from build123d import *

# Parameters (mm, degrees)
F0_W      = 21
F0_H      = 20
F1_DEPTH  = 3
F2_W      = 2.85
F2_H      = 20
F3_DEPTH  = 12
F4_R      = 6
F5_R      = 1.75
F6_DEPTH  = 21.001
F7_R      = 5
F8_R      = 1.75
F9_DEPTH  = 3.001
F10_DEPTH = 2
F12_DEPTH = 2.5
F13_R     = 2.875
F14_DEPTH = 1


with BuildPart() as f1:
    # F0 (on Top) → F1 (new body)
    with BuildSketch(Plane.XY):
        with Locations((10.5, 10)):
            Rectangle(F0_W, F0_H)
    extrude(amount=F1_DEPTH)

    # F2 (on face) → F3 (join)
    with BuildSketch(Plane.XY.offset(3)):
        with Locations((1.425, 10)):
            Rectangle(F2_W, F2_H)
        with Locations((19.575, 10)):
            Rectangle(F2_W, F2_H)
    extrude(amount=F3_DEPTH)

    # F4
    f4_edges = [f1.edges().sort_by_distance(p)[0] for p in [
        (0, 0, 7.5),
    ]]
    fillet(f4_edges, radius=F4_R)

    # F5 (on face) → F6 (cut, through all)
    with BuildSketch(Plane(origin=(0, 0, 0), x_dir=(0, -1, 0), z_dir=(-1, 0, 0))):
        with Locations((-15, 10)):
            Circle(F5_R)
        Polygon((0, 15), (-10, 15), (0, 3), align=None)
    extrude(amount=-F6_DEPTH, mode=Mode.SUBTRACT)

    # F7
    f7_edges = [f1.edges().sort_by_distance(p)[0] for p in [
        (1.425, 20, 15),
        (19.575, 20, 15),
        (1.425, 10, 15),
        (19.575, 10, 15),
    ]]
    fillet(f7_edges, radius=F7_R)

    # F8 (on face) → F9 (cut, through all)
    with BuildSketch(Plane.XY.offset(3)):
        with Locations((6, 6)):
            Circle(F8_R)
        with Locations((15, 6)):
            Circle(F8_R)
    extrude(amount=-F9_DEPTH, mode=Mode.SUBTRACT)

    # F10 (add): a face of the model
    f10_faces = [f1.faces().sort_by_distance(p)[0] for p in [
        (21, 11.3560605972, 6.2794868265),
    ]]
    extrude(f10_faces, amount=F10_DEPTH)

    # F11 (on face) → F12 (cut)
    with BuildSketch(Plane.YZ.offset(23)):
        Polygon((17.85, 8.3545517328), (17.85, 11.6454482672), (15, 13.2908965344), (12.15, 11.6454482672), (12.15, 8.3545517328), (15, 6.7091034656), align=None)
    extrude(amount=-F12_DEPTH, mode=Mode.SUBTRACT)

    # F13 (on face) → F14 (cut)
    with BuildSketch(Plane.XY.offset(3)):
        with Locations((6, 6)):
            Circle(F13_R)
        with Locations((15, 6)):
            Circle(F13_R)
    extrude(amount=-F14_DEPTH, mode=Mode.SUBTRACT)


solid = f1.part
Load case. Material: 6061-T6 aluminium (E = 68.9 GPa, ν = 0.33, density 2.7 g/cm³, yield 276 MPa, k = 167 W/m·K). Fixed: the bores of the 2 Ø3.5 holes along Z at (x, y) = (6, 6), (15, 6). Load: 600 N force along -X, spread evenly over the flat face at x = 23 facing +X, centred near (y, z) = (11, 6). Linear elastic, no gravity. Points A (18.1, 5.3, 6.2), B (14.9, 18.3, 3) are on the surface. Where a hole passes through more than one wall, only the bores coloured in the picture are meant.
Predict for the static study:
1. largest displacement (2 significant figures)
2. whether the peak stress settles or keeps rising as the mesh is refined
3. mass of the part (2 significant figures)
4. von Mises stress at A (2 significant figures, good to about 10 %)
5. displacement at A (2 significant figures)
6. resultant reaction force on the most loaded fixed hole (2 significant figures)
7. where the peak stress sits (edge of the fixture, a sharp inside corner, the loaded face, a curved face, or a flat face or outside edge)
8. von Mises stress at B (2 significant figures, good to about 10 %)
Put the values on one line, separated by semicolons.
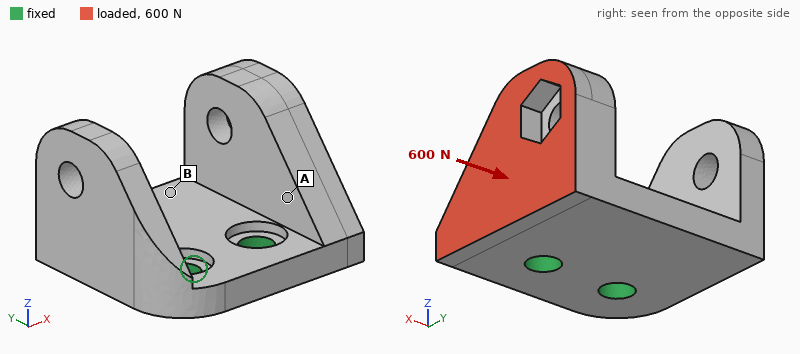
0.11 mm; keeps rising; 6.7 g; 20 MPa; 0.030 mm; 430 N; edge of the fixture; 68 MPa
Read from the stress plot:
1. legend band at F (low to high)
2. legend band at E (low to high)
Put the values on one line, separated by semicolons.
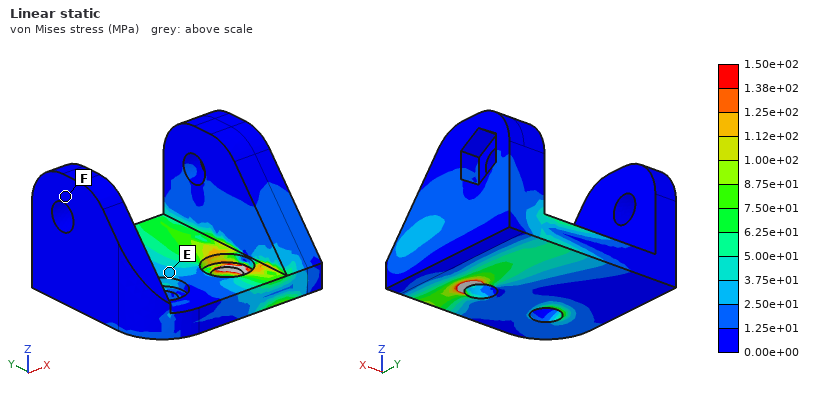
0.00e+00 to 1.25e+01 MPa; 2.50e+01 to 3.75e+01 MPa
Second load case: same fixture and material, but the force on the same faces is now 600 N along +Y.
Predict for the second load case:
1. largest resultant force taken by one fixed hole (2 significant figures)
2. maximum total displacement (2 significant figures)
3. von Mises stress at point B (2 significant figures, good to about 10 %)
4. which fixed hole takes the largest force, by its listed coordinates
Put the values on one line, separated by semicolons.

910 N; 74 µm; 27 MPa; (15, 6)
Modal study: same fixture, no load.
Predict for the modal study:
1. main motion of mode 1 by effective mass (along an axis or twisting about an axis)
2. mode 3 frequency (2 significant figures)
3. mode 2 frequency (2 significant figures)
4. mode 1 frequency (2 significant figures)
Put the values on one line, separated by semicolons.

along Z; 9700 Hz; 8000 Hz; 6900 Hz
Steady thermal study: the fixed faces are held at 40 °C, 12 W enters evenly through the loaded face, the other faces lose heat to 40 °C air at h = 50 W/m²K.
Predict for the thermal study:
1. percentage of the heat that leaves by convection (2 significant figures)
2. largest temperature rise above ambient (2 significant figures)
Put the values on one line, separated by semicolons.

3.8 %; 14 K
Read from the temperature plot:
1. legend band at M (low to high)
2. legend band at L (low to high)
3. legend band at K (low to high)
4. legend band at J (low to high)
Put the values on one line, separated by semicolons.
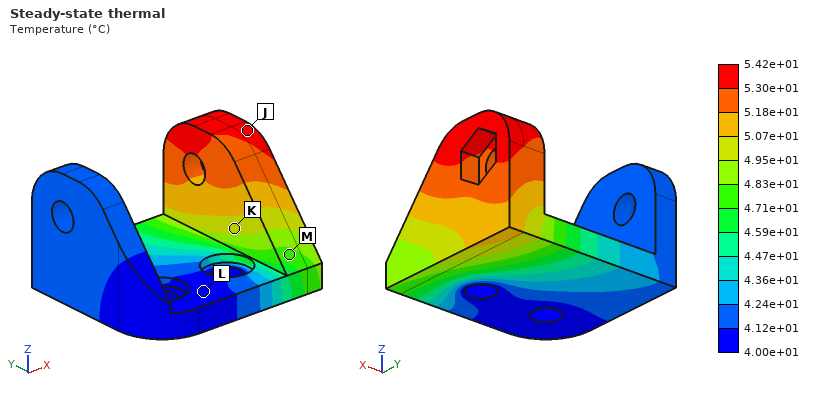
4.71e+01 to 4.83e+01 °C; 4.00e+01 to 4.12e+01 °C; 4.95e+01 to 5.07e+01 °C; 5.30e+01 to 5.42e+01 °C
